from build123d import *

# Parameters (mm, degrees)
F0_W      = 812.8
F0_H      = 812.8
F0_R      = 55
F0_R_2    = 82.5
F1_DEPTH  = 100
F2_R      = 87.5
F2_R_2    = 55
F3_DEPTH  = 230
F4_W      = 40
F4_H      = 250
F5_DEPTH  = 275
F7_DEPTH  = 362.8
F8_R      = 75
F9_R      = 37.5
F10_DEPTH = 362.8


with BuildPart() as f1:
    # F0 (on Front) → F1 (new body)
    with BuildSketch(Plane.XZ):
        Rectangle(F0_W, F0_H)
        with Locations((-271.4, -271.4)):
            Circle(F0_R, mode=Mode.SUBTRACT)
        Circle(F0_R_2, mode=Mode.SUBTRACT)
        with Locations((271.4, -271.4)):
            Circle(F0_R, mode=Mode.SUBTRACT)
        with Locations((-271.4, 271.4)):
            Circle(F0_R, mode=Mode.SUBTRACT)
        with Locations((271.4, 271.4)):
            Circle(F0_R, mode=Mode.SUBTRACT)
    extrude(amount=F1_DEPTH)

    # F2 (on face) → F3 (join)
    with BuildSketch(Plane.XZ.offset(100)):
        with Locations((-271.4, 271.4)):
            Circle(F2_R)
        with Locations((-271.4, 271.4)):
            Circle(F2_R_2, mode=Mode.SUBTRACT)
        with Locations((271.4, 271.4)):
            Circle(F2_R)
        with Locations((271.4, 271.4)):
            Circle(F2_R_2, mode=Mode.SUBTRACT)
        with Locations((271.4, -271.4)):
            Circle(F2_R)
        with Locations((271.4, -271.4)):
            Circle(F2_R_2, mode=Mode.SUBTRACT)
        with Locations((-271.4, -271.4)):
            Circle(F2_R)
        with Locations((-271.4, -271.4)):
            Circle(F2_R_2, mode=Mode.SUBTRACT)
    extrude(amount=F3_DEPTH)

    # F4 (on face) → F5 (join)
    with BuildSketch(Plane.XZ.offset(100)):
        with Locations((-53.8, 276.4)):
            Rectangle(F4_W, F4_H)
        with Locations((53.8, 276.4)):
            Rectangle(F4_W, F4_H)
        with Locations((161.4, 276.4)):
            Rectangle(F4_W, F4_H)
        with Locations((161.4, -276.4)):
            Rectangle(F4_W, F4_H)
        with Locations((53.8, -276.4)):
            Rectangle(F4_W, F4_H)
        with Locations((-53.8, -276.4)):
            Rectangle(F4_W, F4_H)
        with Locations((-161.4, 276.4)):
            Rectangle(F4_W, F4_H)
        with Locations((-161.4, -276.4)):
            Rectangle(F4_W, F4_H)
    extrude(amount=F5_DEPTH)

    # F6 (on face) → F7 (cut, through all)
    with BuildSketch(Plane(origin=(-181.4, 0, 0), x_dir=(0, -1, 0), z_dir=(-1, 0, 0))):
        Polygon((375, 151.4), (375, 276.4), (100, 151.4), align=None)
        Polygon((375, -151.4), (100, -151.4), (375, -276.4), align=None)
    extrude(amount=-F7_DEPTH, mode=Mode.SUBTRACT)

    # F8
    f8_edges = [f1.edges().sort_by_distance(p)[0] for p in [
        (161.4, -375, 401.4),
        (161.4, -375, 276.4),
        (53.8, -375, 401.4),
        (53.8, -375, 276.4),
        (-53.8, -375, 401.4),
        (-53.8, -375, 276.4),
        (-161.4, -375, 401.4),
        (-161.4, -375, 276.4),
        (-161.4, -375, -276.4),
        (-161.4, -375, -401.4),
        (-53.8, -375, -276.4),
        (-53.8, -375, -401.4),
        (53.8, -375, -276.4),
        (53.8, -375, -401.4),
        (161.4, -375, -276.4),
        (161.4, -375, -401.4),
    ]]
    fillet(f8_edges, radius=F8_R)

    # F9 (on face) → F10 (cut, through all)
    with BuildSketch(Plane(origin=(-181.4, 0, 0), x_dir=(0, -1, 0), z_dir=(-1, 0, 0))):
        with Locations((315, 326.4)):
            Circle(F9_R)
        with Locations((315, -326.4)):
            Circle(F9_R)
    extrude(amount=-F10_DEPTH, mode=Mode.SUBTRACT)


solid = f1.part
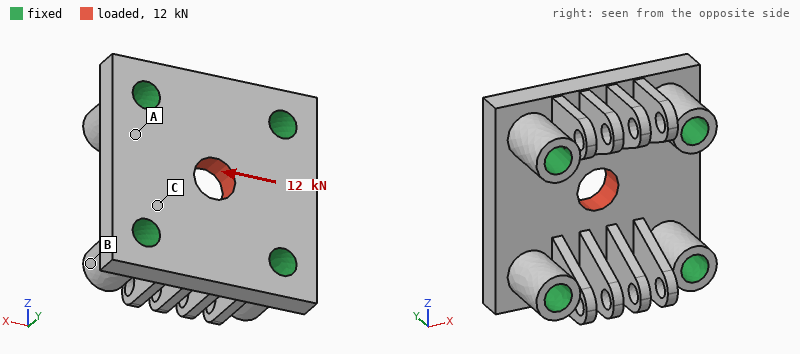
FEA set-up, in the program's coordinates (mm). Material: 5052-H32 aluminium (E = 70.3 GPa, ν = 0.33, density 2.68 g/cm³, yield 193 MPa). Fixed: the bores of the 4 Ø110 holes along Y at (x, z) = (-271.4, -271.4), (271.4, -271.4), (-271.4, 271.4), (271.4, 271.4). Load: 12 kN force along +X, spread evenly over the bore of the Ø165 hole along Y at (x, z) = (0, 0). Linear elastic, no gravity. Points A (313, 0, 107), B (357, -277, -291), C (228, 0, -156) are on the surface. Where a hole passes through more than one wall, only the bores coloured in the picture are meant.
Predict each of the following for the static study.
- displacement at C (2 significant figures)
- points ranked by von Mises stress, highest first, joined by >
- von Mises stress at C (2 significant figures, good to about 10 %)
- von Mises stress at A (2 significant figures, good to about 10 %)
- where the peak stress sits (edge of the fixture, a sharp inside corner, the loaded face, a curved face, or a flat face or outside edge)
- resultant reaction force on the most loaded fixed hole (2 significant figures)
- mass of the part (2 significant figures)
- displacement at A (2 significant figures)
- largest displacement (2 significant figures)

0.29 µm
C > A > B
0.15 MPa
0.084 MPa
a sharp inside corner
3.3 kN
240 kg
0.39 µm
0.90 µm
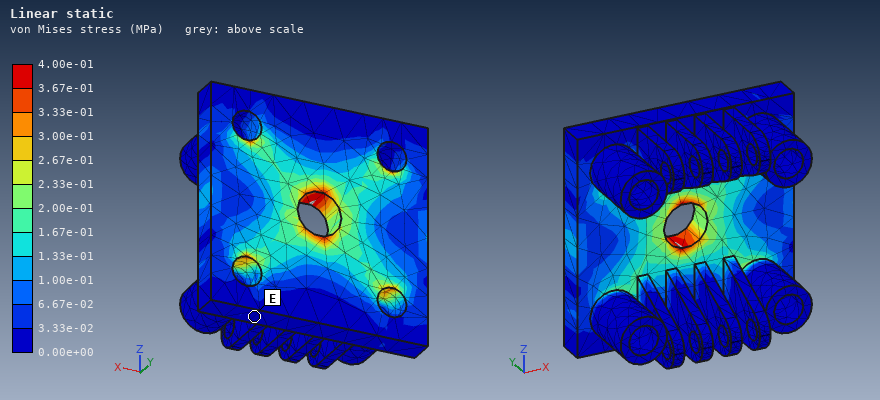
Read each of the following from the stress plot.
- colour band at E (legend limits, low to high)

0.00e+00 to 3.33e-02 MPa
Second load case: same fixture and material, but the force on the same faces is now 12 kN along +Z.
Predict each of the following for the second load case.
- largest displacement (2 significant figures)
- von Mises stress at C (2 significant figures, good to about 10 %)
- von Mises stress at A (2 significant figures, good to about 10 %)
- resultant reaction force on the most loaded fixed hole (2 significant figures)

0.90 µm
0.13 MPa
0.029 MPa
3.3 kN
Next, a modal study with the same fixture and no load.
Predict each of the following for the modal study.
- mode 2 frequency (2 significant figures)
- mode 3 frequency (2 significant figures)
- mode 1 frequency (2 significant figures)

590 Hz
590 Hz
580 Hz
